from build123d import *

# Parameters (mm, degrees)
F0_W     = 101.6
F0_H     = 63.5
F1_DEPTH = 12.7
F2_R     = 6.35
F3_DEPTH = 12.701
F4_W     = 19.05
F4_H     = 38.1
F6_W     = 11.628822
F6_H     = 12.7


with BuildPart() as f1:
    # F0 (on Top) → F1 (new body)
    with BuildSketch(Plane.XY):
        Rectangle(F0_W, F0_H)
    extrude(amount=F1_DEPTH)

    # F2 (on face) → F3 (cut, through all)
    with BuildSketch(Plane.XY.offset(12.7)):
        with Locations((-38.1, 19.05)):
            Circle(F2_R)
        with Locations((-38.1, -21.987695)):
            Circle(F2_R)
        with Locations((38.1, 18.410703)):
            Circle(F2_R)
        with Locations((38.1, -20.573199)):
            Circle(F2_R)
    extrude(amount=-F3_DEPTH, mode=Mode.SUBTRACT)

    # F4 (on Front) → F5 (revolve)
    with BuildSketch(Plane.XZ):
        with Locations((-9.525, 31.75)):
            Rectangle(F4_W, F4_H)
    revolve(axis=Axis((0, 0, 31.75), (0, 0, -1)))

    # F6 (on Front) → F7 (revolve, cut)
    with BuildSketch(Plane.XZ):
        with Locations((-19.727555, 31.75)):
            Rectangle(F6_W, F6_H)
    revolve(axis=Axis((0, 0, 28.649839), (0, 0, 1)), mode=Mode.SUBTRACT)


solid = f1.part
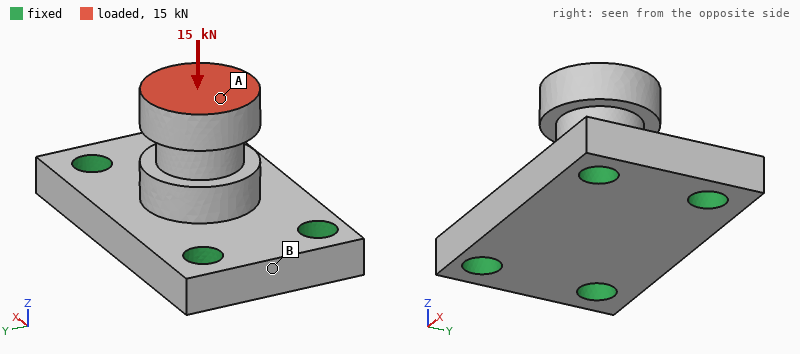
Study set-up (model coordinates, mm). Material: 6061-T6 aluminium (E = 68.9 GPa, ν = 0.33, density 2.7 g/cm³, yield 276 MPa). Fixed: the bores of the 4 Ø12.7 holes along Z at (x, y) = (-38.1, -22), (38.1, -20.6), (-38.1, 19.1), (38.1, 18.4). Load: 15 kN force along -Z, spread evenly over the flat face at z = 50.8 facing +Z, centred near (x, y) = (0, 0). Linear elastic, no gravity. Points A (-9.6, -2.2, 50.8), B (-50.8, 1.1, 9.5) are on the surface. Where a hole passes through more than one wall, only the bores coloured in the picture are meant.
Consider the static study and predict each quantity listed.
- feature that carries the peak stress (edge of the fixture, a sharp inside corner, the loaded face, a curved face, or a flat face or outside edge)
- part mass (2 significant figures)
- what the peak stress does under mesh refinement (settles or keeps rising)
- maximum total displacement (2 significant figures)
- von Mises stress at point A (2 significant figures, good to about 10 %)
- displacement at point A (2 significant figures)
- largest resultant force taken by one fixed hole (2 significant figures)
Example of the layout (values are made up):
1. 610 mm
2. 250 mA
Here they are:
1. edge of the fixture
2. 300 g
3. keeps rising
4. 40 µm
5. 21 MPa
6. 38 µm
7. 4.1 kN
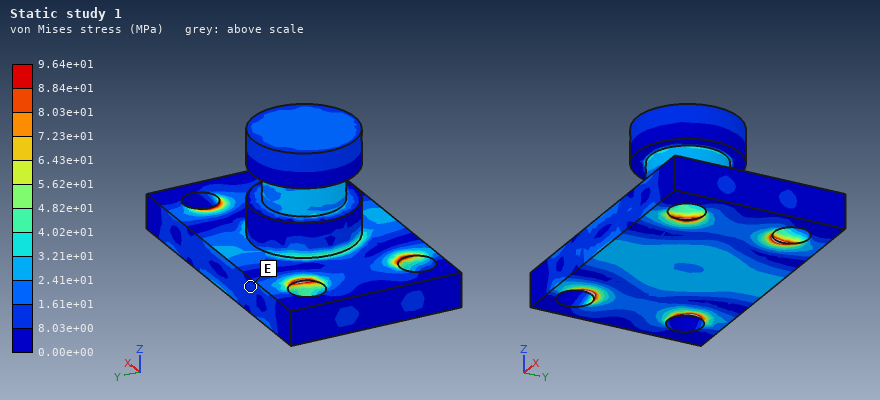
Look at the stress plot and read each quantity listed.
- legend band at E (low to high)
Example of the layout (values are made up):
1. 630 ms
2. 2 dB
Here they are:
1. 8.03e+00 to 1.61e+01 MPa
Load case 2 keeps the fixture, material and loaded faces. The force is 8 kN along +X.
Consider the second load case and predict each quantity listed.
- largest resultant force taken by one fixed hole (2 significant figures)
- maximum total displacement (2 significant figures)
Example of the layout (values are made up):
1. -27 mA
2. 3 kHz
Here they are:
1. 4.1 kN
2. 0.12 mm
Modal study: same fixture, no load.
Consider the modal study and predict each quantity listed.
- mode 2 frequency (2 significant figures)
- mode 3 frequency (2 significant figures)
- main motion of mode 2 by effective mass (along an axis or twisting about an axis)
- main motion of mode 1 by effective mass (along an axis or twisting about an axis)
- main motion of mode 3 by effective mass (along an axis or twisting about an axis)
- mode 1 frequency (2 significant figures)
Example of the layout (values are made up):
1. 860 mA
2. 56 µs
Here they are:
1. 7400 Hz
2. 8600 Hz
3. along X
4. along Y
5. along Z
6. 5800 Hz
